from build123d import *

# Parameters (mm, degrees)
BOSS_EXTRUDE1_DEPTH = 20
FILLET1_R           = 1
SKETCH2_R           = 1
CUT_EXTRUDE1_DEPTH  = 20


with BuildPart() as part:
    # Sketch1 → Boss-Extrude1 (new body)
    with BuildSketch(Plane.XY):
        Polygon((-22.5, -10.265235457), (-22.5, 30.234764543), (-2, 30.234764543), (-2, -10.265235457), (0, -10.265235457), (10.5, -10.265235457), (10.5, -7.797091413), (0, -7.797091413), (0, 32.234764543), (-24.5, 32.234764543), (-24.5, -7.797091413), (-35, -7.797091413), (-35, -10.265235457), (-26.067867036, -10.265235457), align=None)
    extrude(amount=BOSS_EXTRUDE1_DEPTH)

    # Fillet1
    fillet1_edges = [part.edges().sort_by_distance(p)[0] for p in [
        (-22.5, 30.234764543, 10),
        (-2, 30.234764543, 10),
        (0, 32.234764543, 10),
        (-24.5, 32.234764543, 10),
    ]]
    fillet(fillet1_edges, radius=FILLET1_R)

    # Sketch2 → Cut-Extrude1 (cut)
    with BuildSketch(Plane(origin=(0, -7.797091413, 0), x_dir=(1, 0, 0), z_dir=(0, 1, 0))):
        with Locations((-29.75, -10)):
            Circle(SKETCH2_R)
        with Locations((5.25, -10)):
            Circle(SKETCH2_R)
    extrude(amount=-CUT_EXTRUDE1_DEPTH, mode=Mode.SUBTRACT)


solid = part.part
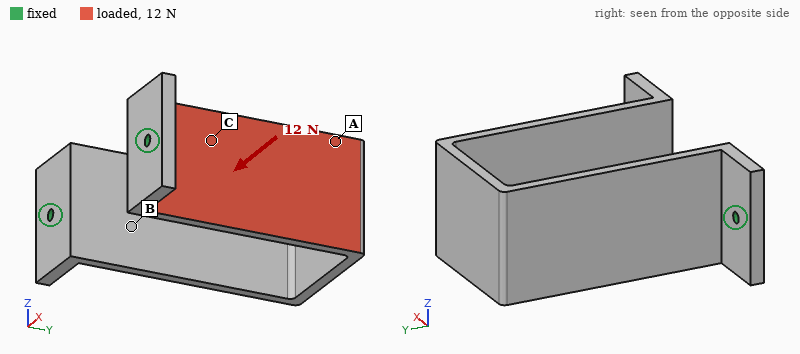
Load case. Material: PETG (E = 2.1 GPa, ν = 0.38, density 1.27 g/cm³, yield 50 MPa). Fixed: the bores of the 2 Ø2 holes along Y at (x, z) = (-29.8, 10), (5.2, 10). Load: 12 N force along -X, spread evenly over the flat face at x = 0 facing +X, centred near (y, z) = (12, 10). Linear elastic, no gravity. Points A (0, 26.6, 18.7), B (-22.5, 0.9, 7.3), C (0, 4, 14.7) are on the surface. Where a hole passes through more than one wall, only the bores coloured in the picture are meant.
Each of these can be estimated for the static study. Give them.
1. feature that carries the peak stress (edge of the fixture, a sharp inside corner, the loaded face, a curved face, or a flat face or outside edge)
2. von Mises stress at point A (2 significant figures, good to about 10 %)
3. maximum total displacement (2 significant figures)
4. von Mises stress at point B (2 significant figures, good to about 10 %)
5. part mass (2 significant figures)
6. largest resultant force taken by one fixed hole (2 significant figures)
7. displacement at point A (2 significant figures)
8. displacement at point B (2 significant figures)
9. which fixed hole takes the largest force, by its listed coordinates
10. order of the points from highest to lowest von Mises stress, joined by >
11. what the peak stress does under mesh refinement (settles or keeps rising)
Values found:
edge of the fixture
3.2 MPa
0.73 mm
1.9 MPa
6.7 g
10.0 N
0.73 mm
0.14 mm
(5.2, 10)
A > B > C
keeps rising
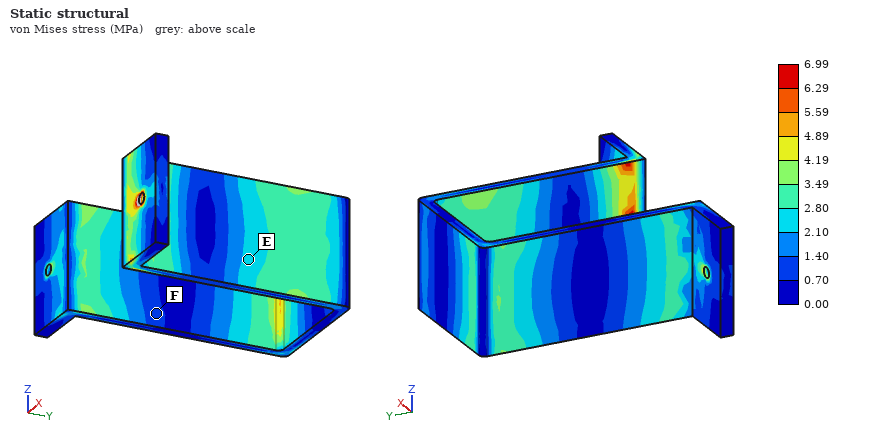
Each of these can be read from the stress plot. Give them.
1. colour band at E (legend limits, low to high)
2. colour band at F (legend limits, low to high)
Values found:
2.10 to 2.80 MPa
0.70 to 1.40 MPa
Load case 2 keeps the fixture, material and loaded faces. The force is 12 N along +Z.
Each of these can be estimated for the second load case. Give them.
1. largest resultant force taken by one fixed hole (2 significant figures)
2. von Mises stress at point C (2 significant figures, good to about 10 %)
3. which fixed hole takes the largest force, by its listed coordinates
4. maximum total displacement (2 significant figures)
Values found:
11 N
1.8 MPa
(5.2, 10)
0.78 mm
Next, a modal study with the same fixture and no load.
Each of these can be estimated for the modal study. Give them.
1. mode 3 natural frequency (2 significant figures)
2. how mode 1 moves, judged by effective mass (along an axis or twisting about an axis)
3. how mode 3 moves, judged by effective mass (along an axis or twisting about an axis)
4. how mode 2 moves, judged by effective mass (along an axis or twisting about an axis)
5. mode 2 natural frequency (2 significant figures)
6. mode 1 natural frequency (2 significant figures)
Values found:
590 Hz
along X
twisting about Y
along Z
340 Hz
290 Hz
